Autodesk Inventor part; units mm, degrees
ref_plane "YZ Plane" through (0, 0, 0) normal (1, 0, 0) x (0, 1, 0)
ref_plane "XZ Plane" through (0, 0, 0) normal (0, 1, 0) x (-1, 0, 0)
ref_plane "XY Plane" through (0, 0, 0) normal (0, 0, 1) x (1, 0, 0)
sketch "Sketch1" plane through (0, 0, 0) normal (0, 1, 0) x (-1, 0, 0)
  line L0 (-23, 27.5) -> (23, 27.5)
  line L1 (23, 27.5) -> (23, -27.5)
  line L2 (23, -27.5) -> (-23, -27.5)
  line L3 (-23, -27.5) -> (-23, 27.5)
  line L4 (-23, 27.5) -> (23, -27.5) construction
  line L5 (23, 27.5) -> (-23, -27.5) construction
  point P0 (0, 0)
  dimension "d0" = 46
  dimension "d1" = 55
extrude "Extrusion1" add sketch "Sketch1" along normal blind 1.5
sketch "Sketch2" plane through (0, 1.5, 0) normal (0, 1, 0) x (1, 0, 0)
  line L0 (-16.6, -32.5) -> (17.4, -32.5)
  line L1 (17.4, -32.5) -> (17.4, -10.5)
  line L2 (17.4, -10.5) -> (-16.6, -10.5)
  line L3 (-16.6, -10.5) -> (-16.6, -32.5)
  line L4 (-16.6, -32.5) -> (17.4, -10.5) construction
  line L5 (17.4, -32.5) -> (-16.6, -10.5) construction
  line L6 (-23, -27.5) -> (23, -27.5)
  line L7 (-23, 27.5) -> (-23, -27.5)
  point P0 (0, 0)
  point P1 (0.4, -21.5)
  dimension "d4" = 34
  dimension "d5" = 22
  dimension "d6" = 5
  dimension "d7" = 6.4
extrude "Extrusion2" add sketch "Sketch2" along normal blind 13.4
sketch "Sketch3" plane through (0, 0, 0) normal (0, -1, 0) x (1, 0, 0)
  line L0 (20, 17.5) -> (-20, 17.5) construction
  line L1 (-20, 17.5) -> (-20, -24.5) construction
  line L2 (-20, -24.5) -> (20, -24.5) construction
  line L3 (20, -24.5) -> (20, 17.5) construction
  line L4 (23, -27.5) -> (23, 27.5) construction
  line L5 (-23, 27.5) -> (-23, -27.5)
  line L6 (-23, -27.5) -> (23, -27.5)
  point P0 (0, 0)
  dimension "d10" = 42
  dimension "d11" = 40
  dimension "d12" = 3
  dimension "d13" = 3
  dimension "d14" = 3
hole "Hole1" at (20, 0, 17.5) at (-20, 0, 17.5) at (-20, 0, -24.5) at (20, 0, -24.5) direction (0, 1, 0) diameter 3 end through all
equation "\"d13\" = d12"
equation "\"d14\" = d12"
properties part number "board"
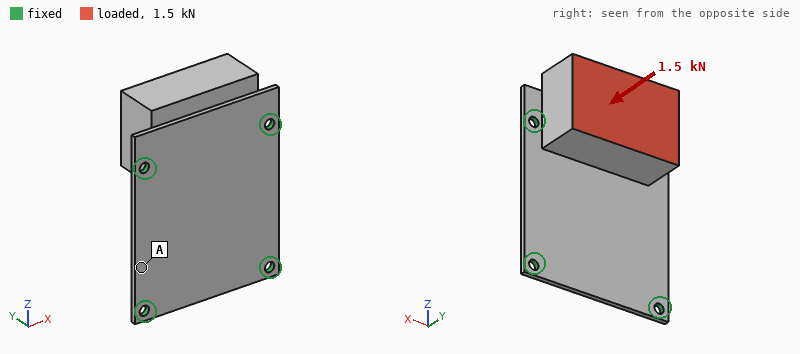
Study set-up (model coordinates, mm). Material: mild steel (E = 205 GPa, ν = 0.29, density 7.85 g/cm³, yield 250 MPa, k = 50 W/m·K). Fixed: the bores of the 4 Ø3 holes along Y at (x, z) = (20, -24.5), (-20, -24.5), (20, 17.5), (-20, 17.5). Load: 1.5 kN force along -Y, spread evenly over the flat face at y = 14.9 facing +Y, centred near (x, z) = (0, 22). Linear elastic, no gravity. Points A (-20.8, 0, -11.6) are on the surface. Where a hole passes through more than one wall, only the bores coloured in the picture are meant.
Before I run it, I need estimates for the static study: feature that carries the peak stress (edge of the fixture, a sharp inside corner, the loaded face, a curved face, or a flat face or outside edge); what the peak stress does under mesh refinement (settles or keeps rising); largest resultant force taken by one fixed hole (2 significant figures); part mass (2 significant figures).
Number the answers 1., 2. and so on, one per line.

1. edge of the fixture
2. keeps rising
3. 900 N
4. 110 g
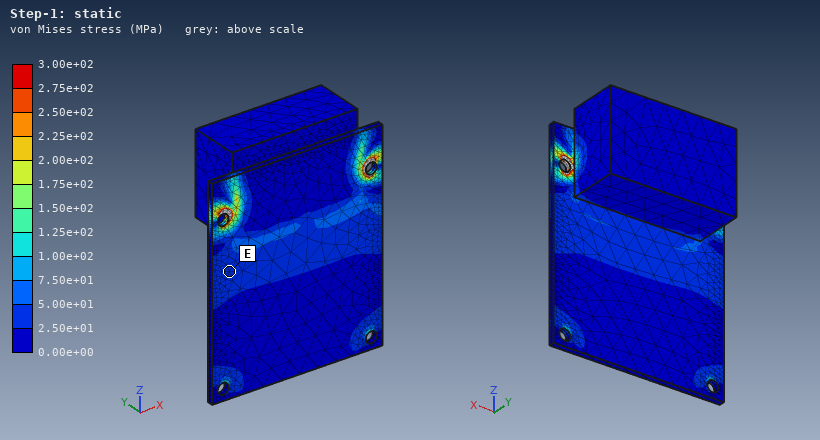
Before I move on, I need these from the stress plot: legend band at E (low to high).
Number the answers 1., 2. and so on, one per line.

1. 2.50e+01 to 5.00e+01 MPa
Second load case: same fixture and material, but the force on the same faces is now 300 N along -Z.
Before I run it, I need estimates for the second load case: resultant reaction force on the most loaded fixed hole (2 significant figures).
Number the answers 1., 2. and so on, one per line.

1. 120 N
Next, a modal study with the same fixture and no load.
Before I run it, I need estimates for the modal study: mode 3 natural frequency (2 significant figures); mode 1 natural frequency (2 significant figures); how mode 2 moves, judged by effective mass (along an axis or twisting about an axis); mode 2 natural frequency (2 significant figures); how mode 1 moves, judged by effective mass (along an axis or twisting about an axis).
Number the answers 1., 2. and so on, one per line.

1. 6500 Hz
2. 2000 Hz
3. along Y
4. 4700 Hz
5. along Z
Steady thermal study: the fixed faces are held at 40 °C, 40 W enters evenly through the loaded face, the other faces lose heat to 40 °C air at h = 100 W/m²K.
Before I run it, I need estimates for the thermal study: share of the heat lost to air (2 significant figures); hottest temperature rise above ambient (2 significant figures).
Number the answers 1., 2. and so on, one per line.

1. 48 %
2. 66 K
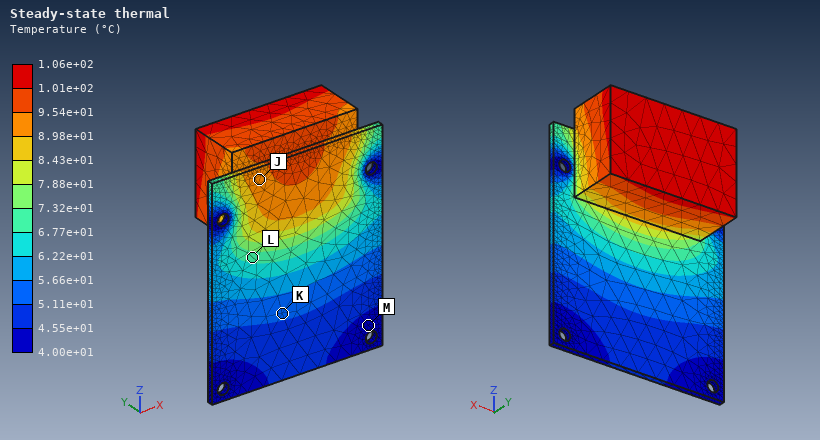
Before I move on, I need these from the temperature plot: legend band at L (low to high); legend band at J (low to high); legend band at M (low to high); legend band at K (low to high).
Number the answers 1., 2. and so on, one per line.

1. 6.77e+01 to 7.32e+01 °C
2. 8.98e+01 to 9.54e+01 °C
3. 4.00e+01 to 4.55e+01 °C
4. 5.11e+01 to 5.66e+01 °C
